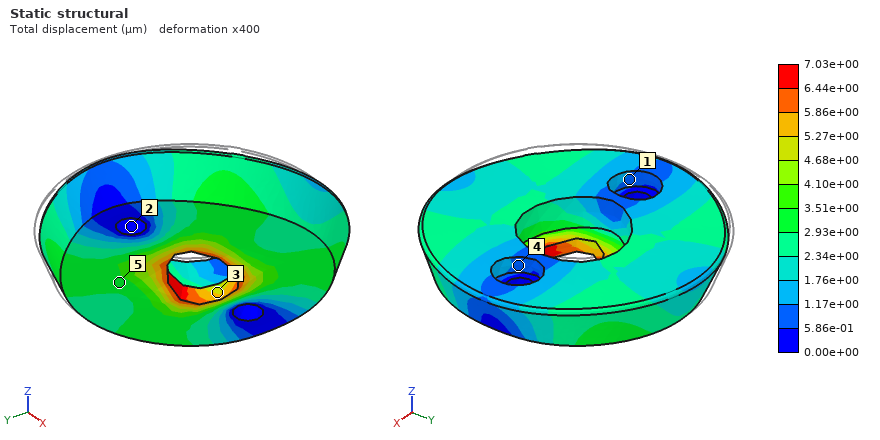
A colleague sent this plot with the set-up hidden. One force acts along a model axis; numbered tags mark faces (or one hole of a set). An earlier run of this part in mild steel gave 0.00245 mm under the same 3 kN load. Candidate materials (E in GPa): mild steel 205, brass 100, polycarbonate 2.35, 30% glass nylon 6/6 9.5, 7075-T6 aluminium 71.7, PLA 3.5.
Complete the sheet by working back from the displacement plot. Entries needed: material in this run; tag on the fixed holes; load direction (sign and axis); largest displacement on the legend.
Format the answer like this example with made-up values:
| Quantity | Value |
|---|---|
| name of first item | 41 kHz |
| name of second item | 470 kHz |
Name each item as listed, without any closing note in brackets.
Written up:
| Quantity | Value |
|---|---|
| material in this run | 7075-T6 aluminium |
| tag on the fixed holes | 2 |
| load direction | +X |
| largest displacement on the legend | 7.03e+00 µm |
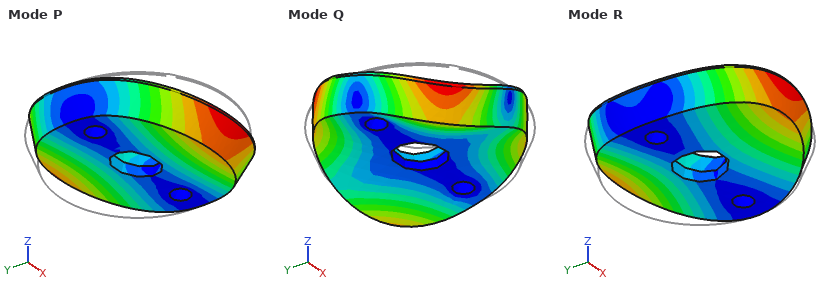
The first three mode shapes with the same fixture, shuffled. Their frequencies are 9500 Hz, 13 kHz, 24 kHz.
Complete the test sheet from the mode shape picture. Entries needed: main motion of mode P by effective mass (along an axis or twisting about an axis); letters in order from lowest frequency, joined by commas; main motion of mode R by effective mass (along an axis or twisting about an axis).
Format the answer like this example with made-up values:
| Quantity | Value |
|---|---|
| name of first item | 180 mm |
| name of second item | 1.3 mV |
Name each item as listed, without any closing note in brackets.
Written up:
| Quantity | Value |
|---|---|
| main motion of mode P by effective mass | twisting about X |
| letters in order from lowest frequency, joined by commas | P, R, Q |
| main motion of mode R by effective mass | along Z |
